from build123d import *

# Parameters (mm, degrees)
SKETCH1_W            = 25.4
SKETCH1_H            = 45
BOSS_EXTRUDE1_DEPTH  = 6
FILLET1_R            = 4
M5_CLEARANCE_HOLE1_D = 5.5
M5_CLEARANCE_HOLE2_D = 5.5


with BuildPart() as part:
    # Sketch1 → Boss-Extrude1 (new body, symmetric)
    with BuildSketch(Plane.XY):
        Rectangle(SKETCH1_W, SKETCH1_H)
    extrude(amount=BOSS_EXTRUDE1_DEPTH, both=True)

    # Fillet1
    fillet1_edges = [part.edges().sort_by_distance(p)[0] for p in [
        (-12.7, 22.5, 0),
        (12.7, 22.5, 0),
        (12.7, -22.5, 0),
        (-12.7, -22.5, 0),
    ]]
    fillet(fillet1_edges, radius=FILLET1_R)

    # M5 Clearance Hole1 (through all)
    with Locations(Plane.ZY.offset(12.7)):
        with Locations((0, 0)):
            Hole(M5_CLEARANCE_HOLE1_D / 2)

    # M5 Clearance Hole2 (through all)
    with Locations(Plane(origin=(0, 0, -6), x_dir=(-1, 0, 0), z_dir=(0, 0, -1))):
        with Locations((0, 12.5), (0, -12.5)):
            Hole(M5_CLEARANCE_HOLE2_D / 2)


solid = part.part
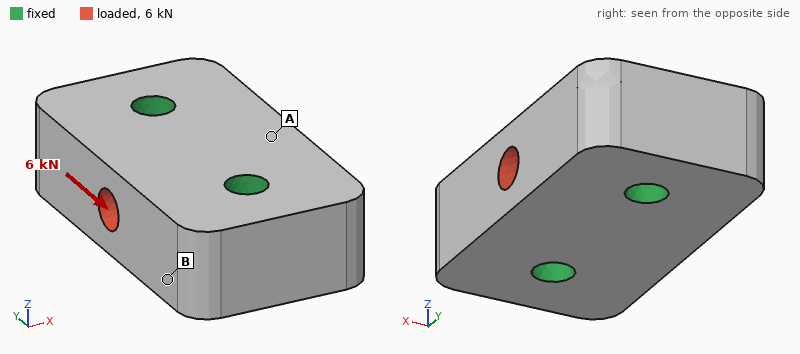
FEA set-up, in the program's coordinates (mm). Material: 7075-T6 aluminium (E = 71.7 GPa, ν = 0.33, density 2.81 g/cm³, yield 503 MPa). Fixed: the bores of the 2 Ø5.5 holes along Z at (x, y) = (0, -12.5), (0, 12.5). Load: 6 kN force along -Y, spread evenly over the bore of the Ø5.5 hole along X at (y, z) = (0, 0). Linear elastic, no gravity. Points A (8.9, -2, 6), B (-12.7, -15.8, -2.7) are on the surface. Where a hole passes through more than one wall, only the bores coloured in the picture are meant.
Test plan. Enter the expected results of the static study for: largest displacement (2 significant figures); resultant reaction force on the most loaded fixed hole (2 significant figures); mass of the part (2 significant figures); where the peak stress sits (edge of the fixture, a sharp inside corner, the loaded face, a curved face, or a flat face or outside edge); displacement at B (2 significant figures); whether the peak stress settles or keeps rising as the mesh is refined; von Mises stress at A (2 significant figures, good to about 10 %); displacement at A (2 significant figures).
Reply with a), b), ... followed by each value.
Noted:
a) 2.9 µm
b) 3.0 kN
c) 35 g
d) edge of the fixture
e) 1.6 µm
f) keeps rising
g) 6.8 MPa
h) 2.0 µm
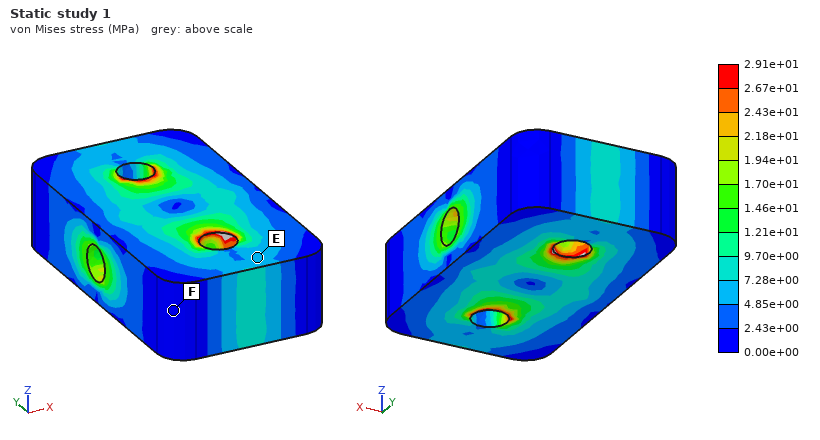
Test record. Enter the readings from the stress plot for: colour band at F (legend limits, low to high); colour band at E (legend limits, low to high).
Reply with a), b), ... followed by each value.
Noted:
a) 0.00e+00 to 2.43e+00 MPa
b) 4.85e+00 to 7.28e+00 MPa
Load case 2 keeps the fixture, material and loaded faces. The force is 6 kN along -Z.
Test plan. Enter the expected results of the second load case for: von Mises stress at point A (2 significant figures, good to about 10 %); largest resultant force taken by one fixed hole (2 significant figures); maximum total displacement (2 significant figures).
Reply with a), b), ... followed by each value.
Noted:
a) 29 MPa
b) 3.0 kN
c) 9.7 µm
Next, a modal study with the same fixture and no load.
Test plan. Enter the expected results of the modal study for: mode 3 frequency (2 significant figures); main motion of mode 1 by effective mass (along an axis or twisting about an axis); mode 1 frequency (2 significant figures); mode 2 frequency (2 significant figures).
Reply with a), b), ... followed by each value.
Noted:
a) 42 kHz
b) twisting about Y
c) 35 kHz
d) 42 kHz
